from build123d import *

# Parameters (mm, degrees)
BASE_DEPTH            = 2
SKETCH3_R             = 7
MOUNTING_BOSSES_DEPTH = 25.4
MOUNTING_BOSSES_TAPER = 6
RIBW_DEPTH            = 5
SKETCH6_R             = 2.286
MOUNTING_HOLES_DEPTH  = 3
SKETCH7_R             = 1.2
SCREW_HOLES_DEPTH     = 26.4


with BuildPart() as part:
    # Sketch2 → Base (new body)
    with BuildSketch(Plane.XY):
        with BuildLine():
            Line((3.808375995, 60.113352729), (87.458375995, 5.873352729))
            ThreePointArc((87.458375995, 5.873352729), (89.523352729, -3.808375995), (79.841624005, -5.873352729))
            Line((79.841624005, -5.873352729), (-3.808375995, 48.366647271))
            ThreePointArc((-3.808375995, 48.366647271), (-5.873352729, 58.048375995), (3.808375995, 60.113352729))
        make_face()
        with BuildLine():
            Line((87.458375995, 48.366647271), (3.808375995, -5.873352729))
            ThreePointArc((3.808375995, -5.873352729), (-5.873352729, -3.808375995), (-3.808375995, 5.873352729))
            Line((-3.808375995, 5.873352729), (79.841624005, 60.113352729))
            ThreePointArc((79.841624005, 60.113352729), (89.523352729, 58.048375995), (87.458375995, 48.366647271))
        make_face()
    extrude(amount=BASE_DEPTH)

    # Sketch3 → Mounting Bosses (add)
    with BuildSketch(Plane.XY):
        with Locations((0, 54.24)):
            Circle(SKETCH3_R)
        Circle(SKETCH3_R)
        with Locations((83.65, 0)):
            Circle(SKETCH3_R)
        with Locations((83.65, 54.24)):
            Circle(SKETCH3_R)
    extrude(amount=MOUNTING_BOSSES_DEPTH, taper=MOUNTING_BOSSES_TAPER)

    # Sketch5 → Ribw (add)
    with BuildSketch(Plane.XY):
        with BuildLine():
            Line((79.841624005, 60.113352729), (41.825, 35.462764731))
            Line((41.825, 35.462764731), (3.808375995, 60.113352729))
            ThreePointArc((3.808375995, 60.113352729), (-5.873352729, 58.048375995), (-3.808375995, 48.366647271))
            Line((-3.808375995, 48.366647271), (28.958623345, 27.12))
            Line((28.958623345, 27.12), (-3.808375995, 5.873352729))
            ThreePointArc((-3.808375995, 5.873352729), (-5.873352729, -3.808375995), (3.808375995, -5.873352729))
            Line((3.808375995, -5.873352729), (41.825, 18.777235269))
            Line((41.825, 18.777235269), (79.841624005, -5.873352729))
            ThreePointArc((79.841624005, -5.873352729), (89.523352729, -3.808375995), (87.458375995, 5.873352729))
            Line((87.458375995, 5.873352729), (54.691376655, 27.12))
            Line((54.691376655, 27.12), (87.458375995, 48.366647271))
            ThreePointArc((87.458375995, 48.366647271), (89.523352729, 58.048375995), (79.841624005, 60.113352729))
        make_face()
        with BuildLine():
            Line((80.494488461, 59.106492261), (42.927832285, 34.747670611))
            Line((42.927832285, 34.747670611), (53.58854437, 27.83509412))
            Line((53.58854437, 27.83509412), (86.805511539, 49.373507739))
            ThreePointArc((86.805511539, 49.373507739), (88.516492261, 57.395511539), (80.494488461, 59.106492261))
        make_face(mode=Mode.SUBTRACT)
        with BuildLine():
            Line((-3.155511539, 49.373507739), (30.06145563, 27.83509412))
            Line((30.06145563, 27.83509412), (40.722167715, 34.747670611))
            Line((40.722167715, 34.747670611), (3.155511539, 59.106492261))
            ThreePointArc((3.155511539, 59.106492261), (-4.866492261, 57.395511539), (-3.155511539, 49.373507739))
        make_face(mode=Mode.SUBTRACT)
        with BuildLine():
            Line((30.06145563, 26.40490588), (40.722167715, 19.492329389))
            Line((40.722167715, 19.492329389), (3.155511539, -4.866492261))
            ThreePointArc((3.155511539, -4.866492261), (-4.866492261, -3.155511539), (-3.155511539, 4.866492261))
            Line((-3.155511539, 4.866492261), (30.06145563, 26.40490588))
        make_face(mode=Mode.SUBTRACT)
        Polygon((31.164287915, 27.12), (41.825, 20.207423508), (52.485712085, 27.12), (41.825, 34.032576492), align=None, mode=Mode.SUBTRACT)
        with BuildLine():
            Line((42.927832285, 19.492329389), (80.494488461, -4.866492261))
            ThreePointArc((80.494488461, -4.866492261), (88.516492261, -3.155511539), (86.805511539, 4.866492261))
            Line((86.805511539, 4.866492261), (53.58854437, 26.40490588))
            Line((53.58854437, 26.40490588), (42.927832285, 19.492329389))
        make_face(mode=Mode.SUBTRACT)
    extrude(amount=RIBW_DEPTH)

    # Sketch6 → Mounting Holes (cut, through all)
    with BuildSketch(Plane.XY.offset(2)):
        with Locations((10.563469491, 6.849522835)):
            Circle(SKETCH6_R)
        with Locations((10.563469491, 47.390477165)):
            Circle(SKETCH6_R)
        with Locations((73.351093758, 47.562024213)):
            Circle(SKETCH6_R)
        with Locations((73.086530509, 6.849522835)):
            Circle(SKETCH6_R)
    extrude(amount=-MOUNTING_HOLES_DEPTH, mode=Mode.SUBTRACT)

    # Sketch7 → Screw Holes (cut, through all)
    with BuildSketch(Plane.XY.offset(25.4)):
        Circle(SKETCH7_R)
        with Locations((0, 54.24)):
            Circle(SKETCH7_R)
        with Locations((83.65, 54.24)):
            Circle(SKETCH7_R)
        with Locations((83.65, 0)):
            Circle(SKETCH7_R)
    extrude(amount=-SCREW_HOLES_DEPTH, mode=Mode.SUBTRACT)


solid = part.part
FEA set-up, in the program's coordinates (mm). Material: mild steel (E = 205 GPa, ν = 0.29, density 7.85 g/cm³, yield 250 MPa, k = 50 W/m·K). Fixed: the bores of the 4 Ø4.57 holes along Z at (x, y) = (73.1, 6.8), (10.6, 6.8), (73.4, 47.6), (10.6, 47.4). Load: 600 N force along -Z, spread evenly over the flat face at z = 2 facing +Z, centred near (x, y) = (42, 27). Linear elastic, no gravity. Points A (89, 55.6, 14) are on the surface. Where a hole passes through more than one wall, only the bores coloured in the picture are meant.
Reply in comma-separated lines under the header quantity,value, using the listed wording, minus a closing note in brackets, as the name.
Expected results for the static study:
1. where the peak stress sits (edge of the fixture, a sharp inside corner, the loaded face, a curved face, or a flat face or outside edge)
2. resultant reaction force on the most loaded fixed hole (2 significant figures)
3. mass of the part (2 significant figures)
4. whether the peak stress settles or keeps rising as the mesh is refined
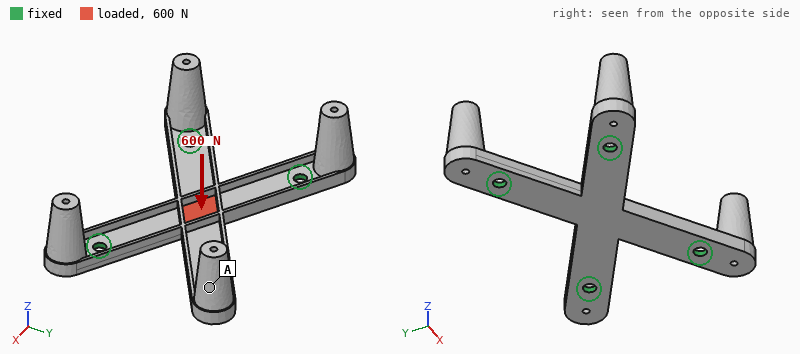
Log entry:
quantity,value
where the peak stress sits,edge of the fixture
resultant reaction force on the most loaded fixed hole,200 N
mass of the part,120 g
whether the peak stress settles or keeps rising as the mesh is refined,keeps rising
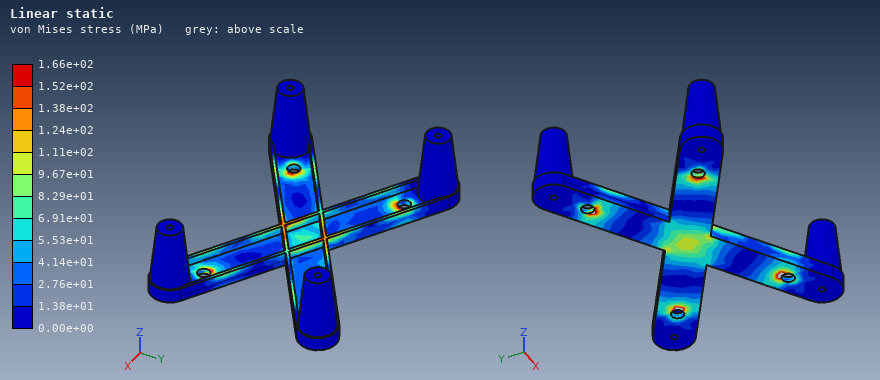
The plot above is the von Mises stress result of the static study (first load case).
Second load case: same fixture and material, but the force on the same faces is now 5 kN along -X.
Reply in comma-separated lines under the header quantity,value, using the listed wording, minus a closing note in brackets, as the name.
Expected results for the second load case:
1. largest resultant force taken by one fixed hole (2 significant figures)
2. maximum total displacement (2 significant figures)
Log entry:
quantity,value
largest resultant force taken by one fixed hole,1.5 kN
maximum total displacement,11 µm
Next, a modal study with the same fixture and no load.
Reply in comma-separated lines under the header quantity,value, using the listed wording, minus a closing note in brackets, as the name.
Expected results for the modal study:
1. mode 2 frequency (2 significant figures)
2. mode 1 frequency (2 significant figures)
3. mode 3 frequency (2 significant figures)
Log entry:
quantity,value
mode 2 frequency,2200 Hz
mode 1 frequency,2100 Hz
mode 3 frequency,2200 Hz
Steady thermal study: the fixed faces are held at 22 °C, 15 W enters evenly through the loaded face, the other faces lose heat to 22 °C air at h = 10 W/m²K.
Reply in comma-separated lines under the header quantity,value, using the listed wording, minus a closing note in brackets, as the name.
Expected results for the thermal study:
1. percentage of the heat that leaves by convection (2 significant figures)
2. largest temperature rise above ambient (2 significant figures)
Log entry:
quantity,value
percentage of the heat that leaves by convection,13 %
largest temperature rise above ambient,75 K
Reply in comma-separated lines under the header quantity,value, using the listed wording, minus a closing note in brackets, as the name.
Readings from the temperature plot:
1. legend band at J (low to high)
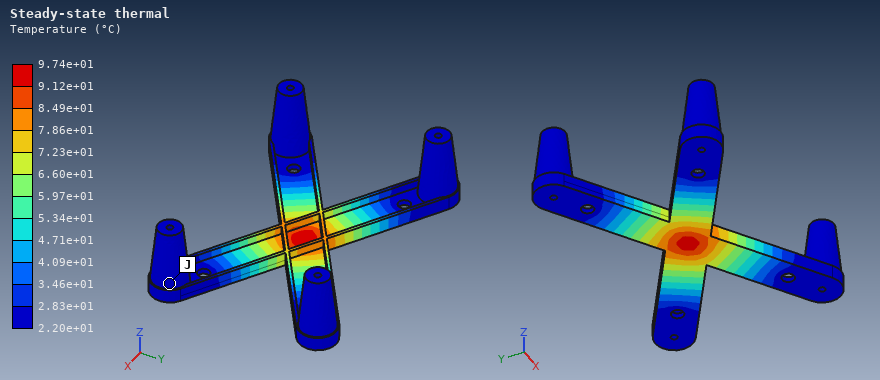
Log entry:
quantity,value
legend band at J,2.20e+01 to 2.83e+01 °C
